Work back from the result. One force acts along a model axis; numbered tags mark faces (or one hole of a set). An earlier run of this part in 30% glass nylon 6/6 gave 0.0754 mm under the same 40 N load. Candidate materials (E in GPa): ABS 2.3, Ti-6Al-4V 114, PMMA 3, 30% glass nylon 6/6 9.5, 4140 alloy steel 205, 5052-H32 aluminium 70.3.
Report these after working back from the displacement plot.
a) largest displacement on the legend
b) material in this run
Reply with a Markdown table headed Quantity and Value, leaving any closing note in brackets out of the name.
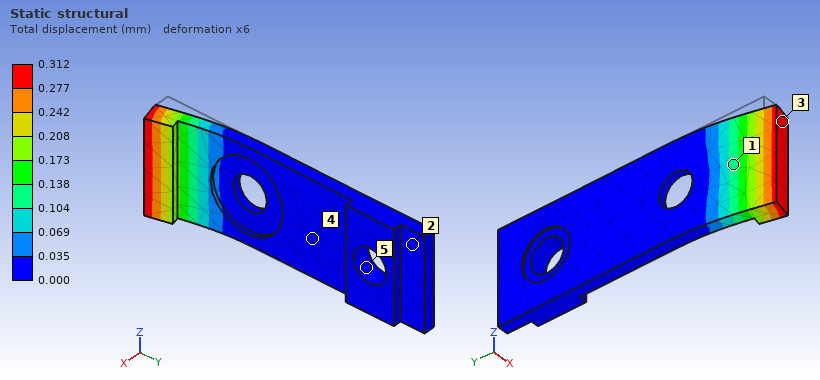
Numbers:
| Quantity | Value |
|---|---|
| largest displacement on the legend | 0.312 mm |
| material in this run | ABS |
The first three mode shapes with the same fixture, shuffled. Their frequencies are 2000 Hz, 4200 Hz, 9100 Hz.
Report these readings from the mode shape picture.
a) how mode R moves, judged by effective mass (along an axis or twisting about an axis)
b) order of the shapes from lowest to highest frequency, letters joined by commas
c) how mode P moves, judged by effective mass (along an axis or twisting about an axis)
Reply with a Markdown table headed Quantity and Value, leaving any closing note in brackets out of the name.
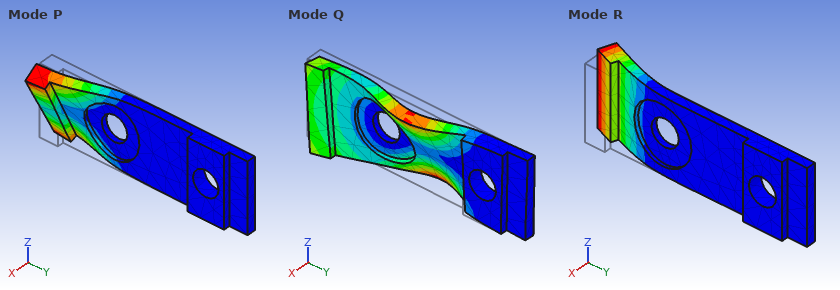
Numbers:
| Quantity | Value |
|---|---|
| how mode R moves, judged by effective mass | along X |
| order of the shapes from lowest to highest frequency, letters joined by commas | R, P, Q |
| how mode P moves, judged by effective mass | twisting about Y |
